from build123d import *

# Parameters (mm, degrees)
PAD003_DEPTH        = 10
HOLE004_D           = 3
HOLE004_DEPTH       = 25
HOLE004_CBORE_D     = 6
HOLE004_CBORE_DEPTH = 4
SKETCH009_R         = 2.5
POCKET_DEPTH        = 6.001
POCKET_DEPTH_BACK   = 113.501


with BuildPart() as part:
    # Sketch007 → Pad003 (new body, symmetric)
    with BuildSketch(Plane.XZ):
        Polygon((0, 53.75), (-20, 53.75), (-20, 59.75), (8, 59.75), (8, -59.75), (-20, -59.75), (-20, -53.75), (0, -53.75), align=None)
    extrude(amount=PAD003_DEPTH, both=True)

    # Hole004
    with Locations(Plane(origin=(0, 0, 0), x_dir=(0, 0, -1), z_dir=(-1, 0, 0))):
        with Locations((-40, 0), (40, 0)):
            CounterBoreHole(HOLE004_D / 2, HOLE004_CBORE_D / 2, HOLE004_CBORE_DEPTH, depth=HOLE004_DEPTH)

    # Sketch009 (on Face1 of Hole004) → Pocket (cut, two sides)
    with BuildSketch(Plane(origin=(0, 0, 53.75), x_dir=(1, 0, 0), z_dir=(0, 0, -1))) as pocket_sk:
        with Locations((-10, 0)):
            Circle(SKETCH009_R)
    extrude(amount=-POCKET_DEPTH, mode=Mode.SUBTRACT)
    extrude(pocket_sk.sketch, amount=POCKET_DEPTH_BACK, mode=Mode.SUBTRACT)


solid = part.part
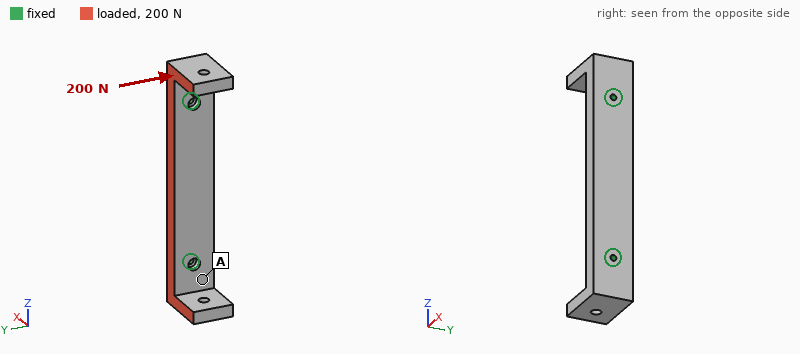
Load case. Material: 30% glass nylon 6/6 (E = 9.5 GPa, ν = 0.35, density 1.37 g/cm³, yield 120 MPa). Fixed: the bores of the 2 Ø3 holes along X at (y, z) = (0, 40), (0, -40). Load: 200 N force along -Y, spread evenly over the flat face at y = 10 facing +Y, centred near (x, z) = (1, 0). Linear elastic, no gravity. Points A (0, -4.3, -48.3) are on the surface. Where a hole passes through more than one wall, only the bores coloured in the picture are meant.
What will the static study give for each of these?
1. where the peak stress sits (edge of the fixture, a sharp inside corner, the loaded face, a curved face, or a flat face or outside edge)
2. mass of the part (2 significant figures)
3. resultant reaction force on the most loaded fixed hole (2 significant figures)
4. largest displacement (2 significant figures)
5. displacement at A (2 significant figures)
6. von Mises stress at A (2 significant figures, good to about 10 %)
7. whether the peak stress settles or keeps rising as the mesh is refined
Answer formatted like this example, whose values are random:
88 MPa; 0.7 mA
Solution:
edge of the fixture; 32 g; 100 N; 47 µm; 11 µm; 1.6 MPa; keeps rising
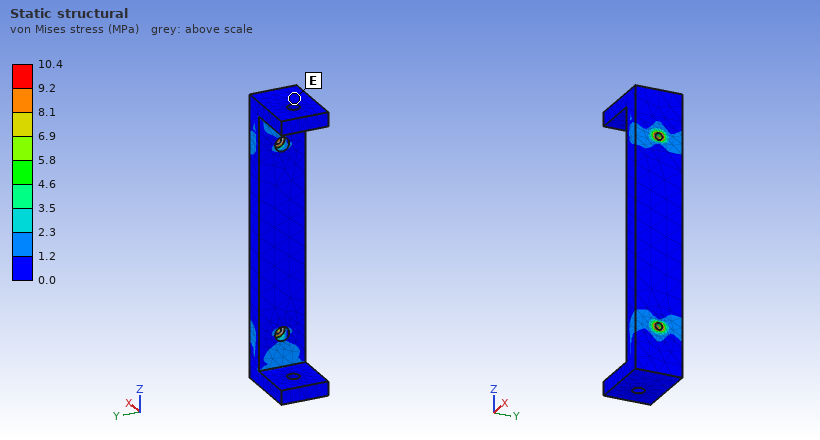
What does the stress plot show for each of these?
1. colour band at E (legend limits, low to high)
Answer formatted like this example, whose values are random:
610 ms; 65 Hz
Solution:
0.0 to 1.2 MPa
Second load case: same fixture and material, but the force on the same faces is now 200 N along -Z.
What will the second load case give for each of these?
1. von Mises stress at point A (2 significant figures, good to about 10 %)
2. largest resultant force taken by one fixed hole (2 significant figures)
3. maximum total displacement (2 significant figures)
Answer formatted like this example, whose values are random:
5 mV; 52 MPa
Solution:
1.2 MPa; 100 N; 50 µm
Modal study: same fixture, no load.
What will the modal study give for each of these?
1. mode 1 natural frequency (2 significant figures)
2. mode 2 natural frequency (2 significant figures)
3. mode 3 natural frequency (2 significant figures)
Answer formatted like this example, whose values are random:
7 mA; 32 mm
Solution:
1800 Hz; 2100 Hz; 2200 Hz
